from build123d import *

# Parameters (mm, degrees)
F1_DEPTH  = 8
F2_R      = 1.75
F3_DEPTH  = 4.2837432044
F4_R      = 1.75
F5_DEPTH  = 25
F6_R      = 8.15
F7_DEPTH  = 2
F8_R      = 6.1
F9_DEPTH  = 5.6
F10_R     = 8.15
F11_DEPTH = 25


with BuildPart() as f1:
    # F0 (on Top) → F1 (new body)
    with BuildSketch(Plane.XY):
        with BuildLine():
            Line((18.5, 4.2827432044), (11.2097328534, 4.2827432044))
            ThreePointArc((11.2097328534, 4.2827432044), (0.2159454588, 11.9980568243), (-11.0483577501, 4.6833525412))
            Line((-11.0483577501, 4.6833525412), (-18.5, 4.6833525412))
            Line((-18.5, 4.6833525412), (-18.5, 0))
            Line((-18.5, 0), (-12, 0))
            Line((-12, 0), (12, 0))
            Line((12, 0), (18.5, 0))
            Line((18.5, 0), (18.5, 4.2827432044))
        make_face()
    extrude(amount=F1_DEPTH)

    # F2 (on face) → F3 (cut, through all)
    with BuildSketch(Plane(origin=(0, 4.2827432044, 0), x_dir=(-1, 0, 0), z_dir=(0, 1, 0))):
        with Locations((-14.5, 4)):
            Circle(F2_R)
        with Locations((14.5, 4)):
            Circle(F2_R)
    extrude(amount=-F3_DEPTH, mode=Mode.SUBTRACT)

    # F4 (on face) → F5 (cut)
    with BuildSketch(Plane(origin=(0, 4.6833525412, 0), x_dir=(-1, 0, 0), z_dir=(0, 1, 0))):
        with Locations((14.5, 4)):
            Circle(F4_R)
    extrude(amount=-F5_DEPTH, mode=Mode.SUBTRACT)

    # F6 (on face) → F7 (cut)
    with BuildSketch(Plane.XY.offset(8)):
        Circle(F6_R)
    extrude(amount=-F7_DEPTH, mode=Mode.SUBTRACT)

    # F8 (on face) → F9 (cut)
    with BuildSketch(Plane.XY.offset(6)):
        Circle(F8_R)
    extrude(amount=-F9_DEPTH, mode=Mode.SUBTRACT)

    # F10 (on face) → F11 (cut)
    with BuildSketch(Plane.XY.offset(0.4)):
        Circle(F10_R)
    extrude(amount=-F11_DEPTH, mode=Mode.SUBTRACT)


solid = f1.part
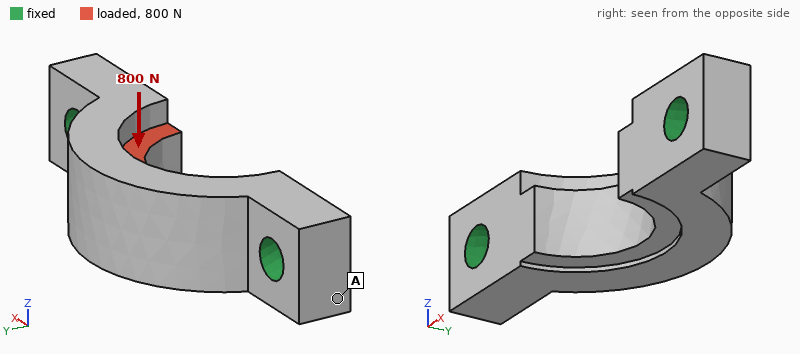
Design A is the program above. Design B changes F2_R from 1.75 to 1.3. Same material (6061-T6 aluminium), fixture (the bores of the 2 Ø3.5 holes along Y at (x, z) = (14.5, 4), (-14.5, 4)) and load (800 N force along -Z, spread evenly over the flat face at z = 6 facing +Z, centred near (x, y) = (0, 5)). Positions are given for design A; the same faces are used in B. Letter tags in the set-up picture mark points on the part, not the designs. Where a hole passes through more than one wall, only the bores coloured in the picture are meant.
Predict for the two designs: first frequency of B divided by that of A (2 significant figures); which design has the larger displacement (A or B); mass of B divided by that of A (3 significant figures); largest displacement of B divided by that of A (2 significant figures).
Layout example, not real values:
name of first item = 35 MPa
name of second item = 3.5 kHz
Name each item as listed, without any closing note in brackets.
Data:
first frequency of B divided by that of A = 0.95
which design has the larger displacement = B
mass of B divided by that of A = 1.01
largest displacement of B divided by that of A = 1.1
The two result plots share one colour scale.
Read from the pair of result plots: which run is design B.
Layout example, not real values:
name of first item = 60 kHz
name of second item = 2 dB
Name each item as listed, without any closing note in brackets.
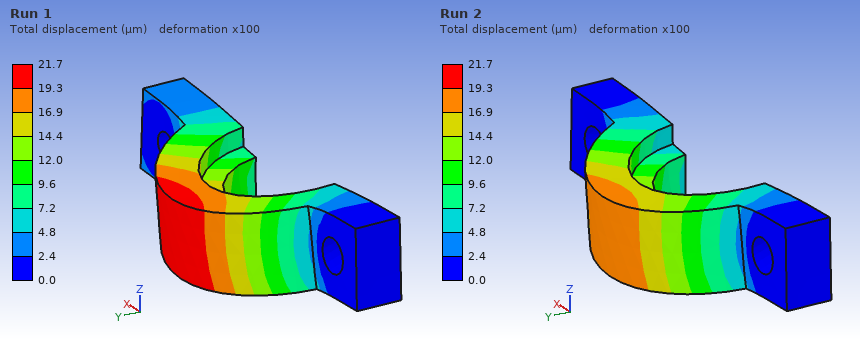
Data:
which run is design B = Run 1
